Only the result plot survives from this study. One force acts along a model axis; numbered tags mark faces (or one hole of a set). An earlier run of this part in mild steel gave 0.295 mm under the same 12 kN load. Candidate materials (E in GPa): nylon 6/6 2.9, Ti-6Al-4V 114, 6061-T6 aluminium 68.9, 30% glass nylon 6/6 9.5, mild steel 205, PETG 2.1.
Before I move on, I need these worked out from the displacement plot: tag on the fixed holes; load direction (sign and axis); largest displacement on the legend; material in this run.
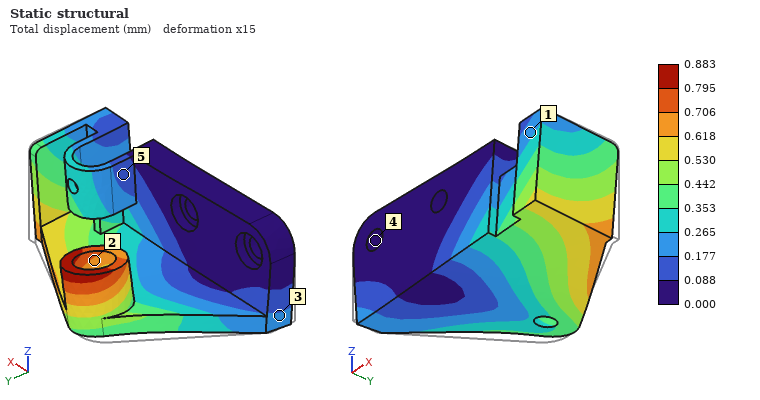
4
+X
0.883 mm
6061-T6 aluminium
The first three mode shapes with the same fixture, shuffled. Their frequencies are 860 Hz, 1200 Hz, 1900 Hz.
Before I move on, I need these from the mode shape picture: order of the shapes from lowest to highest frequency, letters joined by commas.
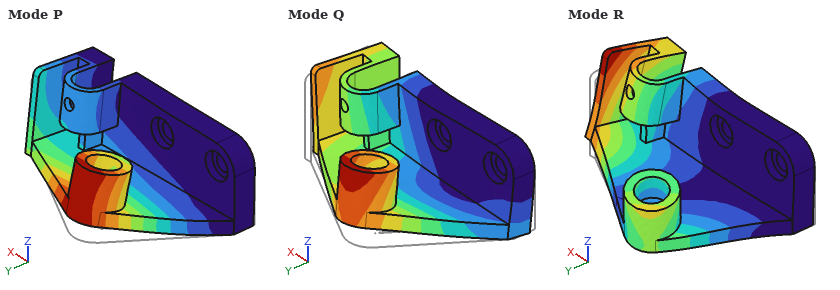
P, Q, R
